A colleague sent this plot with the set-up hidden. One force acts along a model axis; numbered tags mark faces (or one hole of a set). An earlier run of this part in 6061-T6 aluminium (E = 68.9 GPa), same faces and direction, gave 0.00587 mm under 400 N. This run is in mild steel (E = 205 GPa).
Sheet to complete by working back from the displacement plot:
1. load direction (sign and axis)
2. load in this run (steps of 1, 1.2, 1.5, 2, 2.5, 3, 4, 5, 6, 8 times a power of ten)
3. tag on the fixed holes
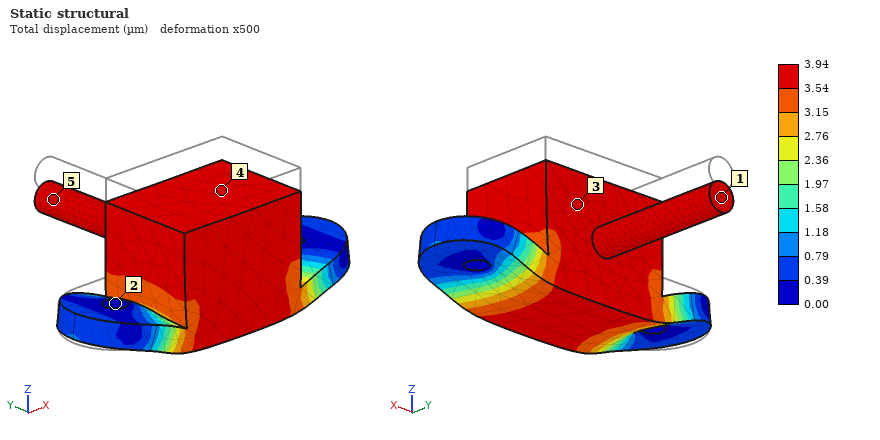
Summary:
-Z
800 N
2
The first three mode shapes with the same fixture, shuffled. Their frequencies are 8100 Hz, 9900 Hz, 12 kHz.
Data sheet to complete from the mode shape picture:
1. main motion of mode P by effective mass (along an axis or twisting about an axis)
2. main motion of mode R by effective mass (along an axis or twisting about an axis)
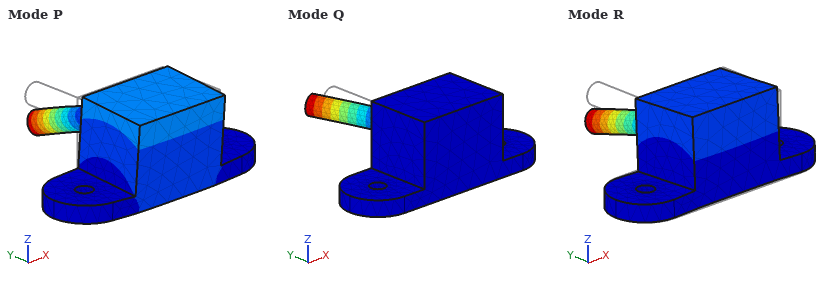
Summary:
along Y
along Y
